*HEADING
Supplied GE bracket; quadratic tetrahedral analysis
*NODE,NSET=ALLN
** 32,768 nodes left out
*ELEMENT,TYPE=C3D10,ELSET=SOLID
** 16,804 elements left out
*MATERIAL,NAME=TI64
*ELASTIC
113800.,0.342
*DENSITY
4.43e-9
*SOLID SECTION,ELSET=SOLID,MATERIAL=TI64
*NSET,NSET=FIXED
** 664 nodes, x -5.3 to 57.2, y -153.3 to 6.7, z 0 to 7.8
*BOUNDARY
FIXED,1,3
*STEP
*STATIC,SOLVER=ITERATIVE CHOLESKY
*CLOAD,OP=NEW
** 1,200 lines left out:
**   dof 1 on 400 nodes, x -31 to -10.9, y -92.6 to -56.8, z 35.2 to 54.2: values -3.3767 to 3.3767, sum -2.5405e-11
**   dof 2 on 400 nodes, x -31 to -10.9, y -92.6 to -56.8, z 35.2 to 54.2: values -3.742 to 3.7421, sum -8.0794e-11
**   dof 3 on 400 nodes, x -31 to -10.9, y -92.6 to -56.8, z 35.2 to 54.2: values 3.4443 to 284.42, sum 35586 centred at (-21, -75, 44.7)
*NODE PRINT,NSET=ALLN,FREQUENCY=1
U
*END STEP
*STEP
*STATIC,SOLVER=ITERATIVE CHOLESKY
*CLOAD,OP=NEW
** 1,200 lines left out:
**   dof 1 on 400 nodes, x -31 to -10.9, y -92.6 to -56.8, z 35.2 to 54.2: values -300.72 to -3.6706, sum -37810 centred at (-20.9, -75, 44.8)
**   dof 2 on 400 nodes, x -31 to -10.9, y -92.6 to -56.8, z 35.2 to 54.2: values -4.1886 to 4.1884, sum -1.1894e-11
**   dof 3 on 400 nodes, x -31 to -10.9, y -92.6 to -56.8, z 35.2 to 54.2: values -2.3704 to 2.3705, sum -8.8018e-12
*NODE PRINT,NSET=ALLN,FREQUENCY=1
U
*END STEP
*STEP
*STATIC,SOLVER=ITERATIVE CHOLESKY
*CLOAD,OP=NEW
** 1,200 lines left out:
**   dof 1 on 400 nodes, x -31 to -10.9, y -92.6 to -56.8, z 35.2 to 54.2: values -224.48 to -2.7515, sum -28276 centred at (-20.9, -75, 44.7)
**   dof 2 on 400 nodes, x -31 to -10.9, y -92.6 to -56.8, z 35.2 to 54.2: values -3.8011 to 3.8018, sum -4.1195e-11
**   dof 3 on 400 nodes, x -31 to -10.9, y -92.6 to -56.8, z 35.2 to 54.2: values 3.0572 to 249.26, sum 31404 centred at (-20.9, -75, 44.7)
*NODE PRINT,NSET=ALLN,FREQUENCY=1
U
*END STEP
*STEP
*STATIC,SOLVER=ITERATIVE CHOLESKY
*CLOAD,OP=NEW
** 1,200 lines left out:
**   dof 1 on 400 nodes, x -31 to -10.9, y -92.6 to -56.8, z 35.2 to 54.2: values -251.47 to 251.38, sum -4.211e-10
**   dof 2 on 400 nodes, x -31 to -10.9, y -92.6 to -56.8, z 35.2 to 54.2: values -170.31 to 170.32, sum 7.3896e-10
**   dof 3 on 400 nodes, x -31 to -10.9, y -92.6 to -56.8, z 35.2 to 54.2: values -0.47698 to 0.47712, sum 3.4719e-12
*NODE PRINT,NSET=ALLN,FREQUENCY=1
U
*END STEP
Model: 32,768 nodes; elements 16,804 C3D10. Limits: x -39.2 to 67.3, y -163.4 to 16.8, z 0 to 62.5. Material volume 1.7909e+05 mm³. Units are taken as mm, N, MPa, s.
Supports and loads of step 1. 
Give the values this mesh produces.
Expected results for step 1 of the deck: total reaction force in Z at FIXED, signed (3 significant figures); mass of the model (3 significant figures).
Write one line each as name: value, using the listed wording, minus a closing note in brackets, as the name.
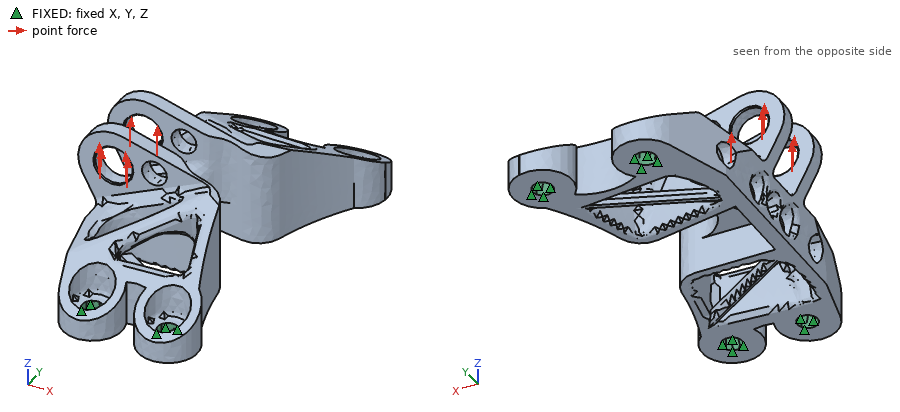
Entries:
total reaction force in Z at FIXED, signed: -35600 N
mass of the model: 0.793 kg
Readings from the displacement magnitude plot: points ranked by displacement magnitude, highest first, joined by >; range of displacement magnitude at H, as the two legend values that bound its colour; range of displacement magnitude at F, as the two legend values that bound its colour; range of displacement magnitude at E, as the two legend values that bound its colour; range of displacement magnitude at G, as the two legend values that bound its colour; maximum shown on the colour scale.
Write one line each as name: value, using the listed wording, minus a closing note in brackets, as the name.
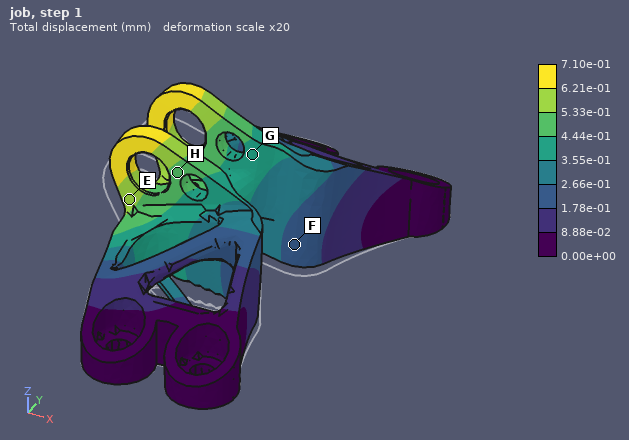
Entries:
points ranked by displacement magnitude, highest first, joined by >: E > H > G > F
range of displacement magnitude at H, as the two legend values that bound its colour: 4.44e-01 to 5.33e-01 mm
range of displacement magnitude at F, as the two legend values that bound its colour: 1.78e-01 to 2.66e-01 mm
range of displacement magnitude at E, as the two legend values that bound its colour: 5.33e-01 to 6.21e-01 mm
range of displacement magnitude at G, as the two legend values that bound its colour: 3.55e-01 to 4.44e-01 mm
maximum shown on the colour scale: 7.10e-01 mm
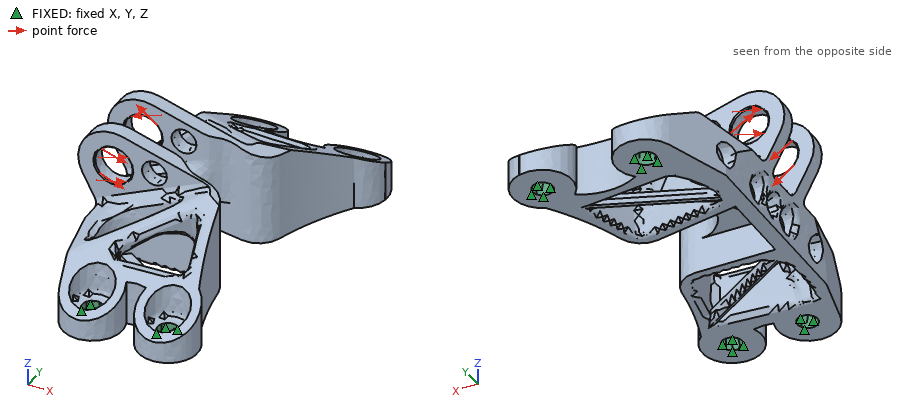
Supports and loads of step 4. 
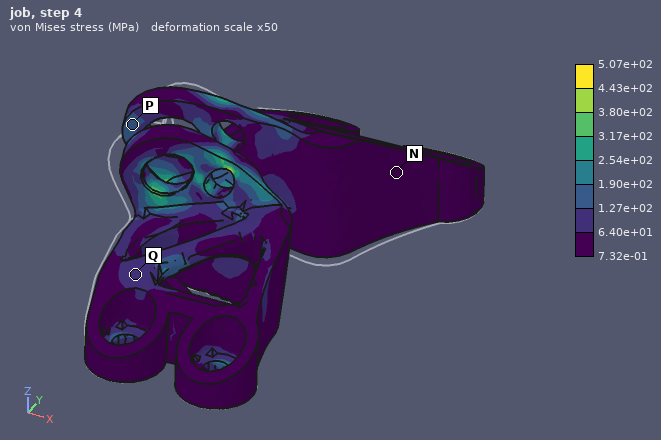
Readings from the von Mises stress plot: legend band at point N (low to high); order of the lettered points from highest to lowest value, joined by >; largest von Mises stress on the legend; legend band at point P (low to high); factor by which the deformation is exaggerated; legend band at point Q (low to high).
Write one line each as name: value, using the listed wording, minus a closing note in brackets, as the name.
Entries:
legend band at point N: 7.32e-01 to 6.40e+01 MPa
order of the lettered points from highest to lowest value, joined by >: P > Q > N
largest von Mises stress on the legend: 5.07e+02 MPa
legend band at point P: 1.27e+02 to 1.90e+02 MPa
factor by which the deformation is exaggerated: 50
legend band at point Q: 6.40e+01 to 1.27e+02 MPa
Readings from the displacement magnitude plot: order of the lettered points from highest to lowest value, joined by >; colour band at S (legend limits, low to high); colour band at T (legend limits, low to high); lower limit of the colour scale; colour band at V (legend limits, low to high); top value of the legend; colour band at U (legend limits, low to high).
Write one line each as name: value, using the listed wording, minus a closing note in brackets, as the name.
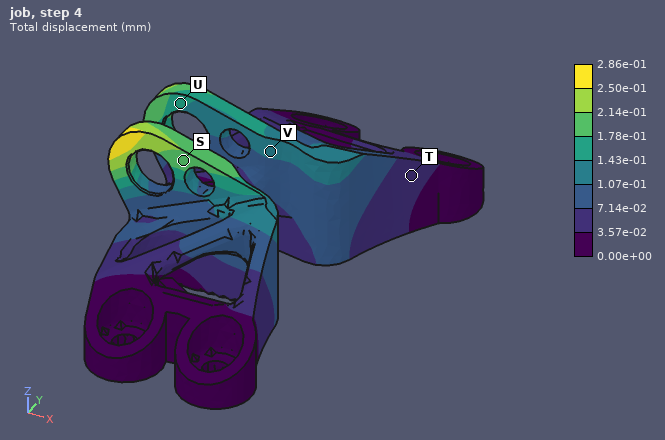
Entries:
order of the lettered points from highest to lowest value, joined by >: S > U > V > T
colour band at S: 1.78e-01 to 2.14e-01 mm
colour band at T: 3.57e-02 to 7.14e-02 mm
lower limit of the colour scale: 0.00e+00 mm
colour band at V: 1.07e-01 to 1.43e-01 mm
top value of the legend: 2.86e-01 mm
colour band at U: 1.43e-01 to 1.78e-01 mm
